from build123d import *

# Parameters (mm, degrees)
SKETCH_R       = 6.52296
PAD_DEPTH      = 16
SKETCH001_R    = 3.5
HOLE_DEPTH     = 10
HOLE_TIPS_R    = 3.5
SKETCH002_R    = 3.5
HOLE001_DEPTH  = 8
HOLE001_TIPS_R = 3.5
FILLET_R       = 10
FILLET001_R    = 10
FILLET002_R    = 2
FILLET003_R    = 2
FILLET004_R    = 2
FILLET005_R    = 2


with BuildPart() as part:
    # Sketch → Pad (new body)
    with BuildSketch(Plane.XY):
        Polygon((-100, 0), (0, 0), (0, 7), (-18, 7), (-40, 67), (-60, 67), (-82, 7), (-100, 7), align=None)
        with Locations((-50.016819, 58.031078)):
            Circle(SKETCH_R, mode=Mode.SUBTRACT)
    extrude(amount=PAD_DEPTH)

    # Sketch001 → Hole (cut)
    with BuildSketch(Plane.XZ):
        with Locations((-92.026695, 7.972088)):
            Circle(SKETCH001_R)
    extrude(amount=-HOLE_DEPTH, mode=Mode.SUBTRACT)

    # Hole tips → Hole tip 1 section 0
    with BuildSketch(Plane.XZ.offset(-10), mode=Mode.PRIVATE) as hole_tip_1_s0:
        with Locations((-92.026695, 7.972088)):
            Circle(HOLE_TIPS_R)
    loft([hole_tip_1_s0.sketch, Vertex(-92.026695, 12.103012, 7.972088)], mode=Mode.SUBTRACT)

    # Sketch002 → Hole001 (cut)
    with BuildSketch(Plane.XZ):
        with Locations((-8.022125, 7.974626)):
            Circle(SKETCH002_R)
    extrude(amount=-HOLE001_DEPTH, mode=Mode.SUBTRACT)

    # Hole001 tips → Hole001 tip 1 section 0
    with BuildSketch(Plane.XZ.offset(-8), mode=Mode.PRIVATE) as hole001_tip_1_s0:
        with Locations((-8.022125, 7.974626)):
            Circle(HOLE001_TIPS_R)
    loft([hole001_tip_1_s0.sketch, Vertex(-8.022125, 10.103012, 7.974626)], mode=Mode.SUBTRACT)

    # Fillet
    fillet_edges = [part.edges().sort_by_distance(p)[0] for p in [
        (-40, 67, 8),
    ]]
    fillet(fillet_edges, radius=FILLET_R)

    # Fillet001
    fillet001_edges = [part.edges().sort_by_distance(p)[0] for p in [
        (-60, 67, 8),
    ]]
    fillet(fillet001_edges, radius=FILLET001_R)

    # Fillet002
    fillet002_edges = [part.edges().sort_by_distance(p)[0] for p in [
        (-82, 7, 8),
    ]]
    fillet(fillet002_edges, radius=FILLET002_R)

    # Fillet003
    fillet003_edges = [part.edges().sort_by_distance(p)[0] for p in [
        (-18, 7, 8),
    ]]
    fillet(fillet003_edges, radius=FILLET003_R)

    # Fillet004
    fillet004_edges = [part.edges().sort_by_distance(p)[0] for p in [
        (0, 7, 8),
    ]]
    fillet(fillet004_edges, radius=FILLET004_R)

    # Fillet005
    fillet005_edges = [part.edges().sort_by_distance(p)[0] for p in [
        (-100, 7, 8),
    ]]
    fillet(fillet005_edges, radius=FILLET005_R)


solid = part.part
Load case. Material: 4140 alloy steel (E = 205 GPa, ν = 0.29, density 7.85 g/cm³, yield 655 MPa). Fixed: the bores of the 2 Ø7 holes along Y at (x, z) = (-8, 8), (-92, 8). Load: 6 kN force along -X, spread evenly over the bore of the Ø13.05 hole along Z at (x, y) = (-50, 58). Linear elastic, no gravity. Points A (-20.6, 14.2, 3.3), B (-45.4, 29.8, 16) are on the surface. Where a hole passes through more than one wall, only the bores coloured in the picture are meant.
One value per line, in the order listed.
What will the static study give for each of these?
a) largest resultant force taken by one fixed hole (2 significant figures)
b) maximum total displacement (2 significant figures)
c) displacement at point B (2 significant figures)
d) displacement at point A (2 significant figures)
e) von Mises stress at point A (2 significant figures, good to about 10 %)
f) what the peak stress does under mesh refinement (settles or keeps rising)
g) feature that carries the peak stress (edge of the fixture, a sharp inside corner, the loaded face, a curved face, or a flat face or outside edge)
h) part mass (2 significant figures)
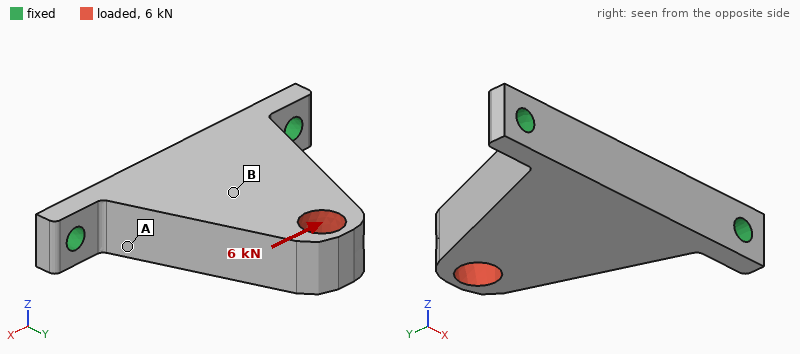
5.6 kN
46 µm
14 µm
13 µm
65 MPa
keeps rising
edge of the fixture
380 g
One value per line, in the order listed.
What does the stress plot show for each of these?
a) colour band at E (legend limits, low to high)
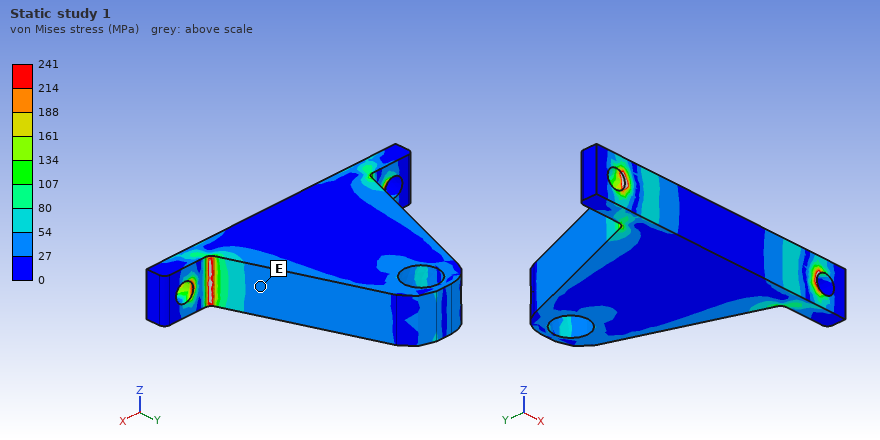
27 to 54 MPa
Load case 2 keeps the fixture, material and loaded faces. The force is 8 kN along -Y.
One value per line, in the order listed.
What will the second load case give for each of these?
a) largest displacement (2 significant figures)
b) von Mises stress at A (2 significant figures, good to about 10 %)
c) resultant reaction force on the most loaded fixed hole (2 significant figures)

22 µm
51 MPa
4.8 kN
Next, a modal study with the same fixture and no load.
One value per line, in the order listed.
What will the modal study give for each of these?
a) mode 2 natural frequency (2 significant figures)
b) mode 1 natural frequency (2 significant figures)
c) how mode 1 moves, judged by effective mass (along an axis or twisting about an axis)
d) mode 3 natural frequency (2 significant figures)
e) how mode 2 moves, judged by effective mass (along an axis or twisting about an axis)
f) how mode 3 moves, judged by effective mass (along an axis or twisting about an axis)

6200 Hz
1400 Hz
along Z
6600 Hz
along Y
along X
